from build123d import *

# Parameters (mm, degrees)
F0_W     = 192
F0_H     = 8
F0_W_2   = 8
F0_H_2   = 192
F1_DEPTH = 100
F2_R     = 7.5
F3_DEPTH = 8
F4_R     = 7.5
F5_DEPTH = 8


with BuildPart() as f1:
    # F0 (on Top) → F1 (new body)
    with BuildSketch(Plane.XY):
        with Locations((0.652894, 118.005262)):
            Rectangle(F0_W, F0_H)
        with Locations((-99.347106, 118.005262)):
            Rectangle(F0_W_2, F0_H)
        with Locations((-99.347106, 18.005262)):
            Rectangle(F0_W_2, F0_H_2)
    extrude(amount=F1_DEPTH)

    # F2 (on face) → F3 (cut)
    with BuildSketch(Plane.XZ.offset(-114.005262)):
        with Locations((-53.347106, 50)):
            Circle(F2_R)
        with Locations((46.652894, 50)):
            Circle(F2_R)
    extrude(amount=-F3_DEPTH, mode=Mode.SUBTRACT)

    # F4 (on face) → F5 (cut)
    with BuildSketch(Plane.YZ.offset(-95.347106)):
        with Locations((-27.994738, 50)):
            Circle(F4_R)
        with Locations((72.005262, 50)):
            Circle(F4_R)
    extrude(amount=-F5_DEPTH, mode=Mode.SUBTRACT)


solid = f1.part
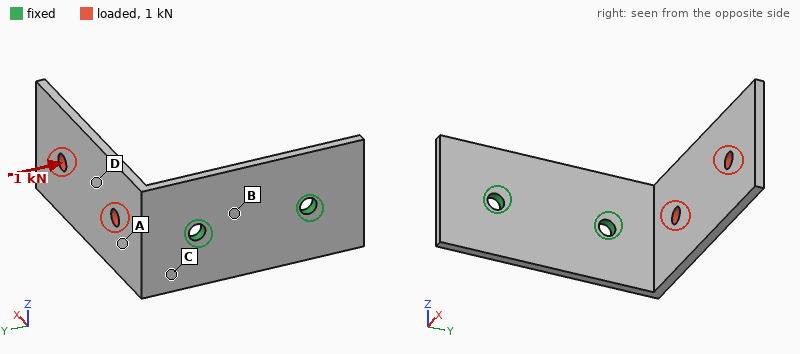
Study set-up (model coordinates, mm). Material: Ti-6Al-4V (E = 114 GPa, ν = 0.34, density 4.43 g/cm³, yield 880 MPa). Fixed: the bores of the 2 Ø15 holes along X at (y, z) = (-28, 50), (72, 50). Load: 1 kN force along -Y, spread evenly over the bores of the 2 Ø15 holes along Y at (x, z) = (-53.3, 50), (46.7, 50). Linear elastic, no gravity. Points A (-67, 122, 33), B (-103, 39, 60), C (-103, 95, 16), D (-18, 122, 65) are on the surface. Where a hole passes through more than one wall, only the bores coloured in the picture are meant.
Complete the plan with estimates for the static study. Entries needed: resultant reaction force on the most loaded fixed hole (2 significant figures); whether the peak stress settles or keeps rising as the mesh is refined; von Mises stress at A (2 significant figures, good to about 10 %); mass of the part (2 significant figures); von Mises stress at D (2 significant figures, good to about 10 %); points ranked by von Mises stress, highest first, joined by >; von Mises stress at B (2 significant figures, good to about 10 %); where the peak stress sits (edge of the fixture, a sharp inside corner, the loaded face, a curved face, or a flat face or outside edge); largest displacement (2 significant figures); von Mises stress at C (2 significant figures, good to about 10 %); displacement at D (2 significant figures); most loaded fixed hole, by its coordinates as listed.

920 N
keeps rising
55 MPa
1.4 kg
29 MPa
C > A > D > B
14 MPa
edge of the fixture
3.4 mm
76 MPa
1.2 mm
(72, 50)
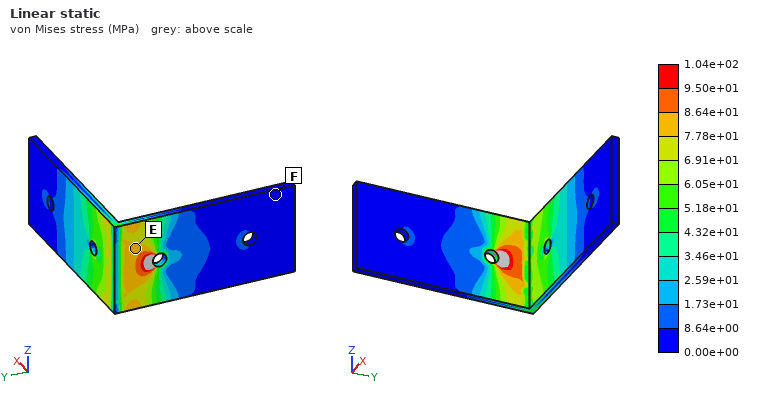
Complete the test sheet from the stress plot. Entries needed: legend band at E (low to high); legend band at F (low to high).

7.78e+01 to 8.64e+01 MPa
0.00e+00 to 8.64e+00 MPa
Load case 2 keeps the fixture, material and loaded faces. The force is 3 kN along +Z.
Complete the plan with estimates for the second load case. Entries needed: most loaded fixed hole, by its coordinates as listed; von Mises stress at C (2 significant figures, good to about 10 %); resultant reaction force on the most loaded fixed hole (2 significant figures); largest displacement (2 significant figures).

(72, 50)
89 MPa
4.1 kN
2.9 mm
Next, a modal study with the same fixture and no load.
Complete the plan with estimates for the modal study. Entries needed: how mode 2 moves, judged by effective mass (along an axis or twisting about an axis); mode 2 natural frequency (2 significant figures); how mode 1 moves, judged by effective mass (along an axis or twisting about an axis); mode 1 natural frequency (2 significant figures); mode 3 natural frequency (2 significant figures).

along Z
230 Hz
along Y
130 Hz
670 Hz
